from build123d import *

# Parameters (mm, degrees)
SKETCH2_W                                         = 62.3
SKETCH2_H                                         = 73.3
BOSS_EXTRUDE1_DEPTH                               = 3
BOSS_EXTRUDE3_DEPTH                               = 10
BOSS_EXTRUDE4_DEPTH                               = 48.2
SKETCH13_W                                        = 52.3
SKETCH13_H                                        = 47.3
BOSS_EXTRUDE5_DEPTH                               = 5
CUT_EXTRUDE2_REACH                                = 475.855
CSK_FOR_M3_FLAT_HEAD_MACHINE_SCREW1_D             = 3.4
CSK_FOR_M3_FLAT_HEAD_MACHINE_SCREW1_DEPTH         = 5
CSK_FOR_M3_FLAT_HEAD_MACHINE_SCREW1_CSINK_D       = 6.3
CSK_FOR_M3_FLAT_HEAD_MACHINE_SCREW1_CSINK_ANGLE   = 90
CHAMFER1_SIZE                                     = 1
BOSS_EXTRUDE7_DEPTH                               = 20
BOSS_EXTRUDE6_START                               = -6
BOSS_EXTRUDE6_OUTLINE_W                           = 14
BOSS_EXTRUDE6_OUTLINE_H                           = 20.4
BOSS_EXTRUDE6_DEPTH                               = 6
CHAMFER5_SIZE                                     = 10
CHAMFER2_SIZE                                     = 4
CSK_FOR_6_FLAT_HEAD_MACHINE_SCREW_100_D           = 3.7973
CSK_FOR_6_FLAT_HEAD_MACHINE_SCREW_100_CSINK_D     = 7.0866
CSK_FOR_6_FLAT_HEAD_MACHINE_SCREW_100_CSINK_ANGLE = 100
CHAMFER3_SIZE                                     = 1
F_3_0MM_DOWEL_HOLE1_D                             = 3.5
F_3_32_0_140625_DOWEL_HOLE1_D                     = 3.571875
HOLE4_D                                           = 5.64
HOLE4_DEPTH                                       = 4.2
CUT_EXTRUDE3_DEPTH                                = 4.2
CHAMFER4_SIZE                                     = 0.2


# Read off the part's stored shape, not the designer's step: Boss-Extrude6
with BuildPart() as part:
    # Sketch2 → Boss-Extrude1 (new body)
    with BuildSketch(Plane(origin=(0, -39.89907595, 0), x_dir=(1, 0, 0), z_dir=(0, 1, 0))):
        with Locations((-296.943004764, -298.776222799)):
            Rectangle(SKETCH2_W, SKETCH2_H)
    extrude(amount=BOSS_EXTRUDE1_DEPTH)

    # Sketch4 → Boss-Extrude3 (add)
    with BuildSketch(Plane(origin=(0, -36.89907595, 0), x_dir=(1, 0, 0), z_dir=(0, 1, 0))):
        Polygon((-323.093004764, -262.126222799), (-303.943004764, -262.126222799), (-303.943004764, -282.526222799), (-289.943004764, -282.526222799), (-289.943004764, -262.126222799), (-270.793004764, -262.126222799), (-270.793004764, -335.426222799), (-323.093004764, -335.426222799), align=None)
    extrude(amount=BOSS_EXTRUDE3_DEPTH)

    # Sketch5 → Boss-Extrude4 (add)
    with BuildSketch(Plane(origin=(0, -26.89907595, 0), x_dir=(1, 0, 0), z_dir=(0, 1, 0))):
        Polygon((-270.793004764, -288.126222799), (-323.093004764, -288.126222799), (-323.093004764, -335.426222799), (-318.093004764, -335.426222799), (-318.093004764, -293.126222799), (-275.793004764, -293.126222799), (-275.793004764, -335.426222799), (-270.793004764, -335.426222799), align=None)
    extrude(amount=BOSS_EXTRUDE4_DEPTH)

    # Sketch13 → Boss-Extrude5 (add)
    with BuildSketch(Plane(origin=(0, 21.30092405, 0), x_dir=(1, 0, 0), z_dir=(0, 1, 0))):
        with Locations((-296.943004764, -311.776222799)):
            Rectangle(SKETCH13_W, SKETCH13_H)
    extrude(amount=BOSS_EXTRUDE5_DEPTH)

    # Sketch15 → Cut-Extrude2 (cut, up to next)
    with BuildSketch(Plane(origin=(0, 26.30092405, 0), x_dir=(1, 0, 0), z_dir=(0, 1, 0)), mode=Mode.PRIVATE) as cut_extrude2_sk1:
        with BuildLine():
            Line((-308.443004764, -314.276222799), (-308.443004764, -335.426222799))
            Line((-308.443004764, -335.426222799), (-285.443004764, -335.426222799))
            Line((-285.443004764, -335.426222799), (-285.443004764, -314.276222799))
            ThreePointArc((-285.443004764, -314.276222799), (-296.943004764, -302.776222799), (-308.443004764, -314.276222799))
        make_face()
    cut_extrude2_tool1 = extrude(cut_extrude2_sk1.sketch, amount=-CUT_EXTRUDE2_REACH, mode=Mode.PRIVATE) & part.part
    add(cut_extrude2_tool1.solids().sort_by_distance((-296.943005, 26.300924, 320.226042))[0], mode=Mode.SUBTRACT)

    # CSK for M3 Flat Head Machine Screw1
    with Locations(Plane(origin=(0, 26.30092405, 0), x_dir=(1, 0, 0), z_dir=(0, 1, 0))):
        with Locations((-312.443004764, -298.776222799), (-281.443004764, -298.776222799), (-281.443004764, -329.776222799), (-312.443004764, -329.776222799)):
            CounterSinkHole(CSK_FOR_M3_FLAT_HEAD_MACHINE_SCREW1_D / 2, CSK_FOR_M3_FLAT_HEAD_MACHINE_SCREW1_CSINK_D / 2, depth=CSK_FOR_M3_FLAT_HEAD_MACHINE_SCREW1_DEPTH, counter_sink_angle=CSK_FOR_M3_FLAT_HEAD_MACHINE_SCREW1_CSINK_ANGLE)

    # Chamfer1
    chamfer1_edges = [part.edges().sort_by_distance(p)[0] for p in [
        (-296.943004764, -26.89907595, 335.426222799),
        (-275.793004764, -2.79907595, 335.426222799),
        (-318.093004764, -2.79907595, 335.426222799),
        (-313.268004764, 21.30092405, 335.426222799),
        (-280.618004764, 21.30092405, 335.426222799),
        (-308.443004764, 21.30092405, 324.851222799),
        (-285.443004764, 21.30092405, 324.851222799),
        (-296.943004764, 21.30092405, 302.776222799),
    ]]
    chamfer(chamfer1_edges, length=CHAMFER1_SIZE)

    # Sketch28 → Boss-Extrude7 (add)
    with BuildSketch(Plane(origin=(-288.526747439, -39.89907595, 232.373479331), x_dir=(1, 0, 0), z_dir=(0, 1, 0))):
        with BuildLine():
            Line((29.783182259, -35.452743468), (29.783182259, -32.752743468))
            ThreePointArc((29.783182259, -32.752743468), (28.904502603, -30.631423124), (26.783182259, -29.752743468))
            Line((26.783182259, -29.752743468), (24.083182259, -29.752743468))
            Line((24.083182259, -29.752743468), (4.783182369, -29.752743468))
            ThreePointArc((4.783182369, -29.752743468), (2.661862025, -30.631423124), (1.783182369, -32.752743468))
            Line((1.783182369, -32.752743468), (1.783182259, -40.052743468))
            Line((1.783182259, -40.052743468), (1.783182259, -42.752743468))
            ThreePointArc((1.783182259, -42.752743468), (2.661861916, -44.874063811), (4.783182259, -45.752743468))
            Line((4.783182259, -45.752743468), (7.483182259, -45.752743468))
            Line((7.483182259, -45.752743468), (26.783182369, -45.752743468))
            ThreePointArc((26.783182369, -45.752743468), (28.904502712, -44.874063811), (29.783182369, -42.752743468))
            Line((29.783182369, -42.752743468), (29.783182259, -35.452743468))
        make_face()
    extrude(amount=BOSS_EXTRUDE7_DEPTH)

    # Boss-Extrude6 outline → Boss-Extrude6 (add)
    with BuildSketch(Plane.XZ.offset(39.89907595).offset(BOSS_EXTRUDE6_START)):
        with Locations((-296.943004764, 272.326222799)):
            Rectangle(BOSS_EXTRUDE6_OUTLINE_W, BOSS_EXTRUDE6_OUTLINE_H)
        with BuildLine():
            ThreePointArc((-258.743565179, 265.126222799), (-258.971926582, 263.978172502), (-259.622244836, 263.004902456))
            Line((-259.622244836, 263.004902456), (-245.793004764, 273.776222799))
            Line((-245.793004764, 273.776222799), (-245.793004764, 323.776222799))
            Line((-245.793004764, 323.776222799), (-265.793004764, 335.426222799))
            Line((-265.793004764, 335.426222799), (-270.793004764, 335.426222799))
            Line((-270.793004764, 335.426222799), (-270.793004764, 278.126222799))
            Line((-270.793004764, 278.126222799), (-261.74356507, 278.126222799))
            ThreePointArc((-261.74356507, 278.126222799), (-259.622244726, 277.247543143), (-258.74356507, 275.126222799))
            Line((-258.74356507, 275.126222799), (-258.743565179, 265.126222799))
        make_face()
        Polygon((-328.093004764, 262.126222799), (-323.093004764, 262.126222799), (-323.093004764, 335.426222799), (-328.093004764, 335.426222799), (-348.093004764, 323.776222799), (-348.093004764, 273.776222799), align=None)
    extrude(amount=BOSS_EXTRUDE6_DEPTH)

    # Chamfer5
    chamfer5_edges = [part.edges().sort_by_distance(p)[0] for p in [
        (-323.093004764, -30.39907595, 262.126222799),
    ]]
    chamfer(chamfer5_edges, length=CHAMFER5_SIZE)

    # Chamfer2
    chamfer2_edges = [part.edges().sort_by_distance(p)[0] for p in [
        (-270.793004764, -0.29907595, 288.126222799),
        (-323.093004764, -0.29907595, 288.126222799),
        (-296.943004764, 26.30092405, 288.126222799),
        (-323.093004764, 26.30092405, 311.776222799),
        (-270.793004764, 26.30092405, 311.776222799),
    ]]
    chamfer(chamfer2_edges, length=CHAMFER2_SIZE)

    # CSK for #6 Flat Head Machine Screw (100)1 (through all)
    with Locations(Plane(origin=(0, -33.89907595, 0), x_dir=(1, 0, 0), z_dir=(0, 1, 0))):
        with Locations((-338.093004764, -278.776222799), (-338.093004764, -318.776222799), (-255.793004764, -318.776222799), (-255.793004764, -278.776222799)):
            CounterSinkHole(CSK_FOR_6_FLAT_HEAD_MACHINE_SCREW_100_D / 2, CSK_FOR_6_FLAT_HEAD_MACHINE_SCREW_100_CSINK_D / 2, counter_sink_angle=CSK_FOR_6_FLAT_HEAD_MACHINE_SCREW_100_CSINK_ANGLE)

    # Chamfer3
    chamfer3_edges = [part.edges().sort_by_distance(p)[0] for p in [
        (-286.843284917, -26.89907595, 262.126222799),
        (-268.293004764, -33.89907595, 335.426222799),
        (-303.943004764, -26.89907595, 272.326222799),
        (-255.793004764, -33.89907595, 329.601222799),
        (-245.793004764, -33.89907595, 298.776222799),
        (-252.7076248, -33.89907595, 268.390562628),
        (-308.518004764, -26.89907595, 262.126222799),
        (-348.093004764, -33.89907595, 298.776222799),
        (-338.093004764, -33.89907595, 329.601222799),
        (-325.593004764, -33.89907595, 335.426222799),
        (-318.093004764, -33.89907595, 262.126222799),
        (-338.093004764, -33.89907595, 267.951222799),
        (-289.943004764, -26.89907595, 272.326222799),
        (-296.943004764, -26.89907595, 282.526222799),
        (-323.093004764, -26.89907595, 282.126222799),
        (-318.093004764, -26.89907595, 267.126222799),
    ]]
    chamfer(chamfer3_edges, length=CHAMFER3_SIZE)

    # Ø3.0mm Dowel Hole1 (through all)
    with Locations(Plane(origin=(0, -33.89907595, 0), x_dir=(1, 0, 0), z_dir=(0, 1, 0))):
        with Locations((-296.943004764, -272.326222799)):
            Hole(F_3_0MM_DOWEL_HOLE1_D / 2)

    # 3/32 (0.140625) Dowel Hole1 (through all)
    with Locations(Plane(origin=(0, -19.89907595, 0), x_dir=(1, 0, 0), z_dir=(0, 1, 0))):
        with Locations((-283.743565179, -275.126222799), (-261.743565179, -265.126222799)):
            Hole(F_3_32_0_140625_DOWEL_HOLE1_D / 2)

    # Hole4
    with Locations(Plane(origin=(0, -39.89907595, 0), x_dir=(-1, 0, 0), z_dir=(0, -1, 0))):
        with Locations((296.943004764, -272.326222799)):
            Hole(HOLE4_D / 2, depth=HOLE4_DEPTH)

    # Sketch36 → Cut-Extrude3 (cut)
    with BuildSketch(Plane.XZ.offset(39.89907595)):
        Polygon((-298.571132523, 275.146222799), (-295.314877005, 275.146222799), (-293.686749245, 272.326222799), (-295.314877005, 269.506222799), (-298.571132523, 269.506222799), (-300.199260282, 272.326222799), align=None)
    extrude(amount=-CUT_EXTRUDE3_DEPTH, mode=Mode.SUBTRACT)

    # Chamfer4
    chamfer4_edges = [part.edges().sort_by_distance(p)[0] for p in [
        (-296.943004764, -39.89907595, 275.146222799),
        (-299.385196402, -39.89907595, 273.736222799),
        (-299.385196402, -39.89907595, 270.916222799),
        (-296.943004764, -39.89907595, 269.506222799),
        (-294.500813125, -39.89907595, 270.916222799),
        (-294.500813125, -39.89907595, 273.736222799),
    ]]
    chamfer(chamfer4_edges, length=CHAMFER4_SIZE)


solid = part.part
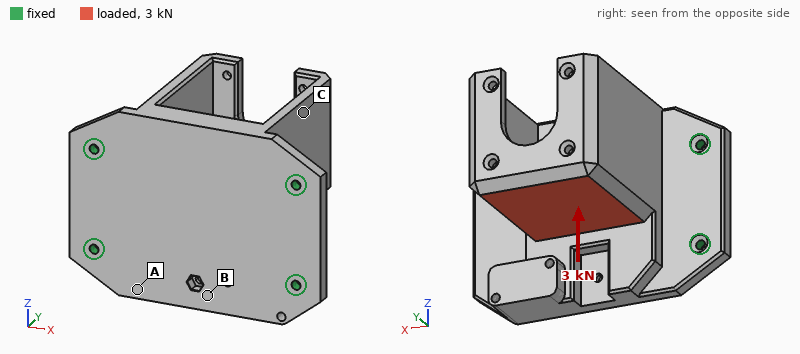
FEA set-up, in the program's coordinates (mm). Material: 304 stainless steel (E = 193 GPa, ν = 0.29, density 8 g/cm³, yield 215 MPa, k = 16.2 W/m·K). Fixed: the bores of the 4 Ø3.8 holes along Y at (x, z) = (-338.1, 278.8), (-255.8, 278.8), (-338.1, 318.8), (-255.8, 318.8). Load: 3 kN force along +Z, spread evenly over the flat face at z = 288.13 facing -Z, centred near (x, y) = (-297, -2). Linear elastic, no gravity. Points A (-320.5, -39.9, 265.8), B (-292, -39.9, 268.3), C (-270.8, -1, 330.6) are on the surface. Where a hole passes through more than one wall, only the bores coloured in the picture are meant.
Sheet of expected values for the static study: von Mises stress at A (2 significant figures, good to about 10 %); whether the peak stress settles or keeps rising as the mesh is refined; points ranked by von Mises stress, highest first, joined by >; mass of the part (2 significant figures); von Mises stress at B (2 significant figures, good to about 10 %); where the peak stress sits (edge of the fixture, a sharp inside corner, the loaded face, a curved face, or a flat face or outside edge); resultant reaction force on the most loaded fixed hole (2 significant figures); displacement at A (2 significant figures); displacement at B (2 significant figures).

27 MPa
keeps rising
A > B > C
880 g
16 MPa
edge of the fixture
1.8 kN
16 µm
18 µm
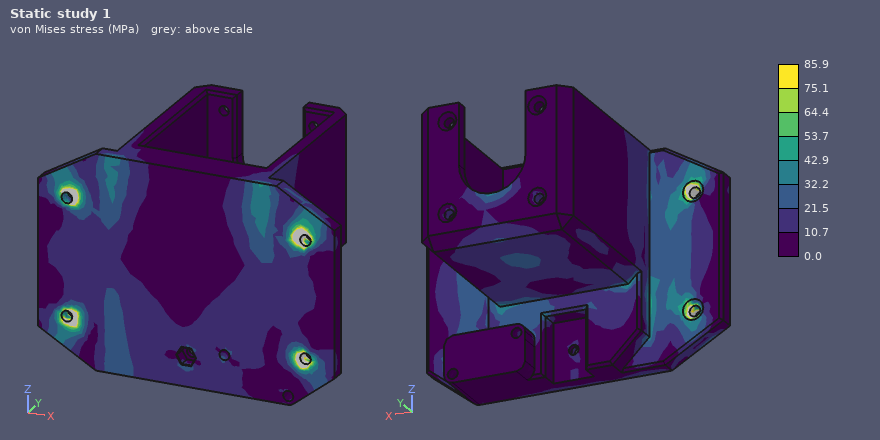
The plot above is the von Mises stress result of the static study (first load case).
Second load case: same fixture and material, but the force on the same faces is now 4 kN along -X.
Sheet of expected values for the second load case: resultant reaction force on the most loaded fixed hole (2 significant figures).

1.7 kN
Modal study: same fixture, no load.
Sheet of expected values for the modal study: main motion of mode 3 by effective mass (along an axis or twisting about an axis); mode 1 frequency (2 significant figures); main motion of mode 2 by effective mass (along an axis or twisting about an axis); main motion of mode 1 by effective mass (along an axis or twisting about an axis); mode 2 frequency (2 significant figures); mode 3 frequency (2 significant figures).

along Y
2200 Hz
along X
along Z
2600 Hz
3500 Hz
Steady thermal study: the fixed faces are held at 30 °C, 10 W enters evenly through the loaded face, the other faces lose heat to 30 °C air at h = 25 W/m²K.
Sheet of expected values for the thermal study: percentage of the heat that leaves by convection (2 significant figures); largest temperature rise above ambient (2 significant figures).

70 %
26 K
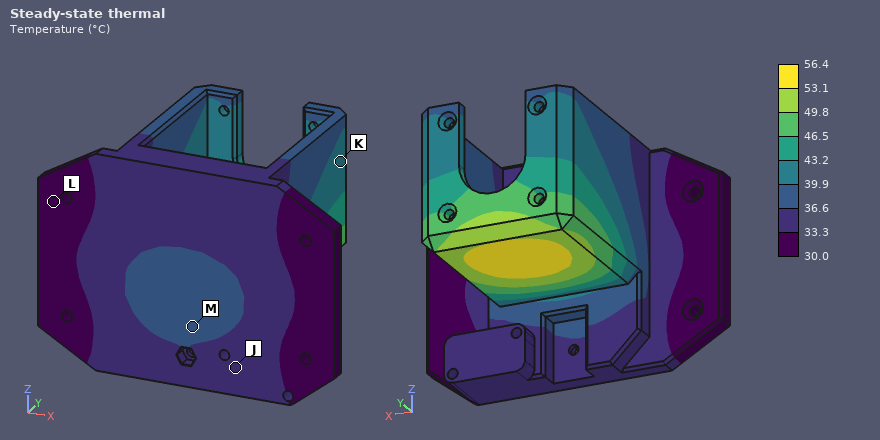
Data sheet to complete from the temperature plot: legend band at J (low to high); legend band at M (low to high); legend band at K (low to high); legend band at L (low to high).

33.3 to 36.6 °C
36.6 to 39.9 °C
39.9 to 43.2 °C
30.0 to 33.3 °C
